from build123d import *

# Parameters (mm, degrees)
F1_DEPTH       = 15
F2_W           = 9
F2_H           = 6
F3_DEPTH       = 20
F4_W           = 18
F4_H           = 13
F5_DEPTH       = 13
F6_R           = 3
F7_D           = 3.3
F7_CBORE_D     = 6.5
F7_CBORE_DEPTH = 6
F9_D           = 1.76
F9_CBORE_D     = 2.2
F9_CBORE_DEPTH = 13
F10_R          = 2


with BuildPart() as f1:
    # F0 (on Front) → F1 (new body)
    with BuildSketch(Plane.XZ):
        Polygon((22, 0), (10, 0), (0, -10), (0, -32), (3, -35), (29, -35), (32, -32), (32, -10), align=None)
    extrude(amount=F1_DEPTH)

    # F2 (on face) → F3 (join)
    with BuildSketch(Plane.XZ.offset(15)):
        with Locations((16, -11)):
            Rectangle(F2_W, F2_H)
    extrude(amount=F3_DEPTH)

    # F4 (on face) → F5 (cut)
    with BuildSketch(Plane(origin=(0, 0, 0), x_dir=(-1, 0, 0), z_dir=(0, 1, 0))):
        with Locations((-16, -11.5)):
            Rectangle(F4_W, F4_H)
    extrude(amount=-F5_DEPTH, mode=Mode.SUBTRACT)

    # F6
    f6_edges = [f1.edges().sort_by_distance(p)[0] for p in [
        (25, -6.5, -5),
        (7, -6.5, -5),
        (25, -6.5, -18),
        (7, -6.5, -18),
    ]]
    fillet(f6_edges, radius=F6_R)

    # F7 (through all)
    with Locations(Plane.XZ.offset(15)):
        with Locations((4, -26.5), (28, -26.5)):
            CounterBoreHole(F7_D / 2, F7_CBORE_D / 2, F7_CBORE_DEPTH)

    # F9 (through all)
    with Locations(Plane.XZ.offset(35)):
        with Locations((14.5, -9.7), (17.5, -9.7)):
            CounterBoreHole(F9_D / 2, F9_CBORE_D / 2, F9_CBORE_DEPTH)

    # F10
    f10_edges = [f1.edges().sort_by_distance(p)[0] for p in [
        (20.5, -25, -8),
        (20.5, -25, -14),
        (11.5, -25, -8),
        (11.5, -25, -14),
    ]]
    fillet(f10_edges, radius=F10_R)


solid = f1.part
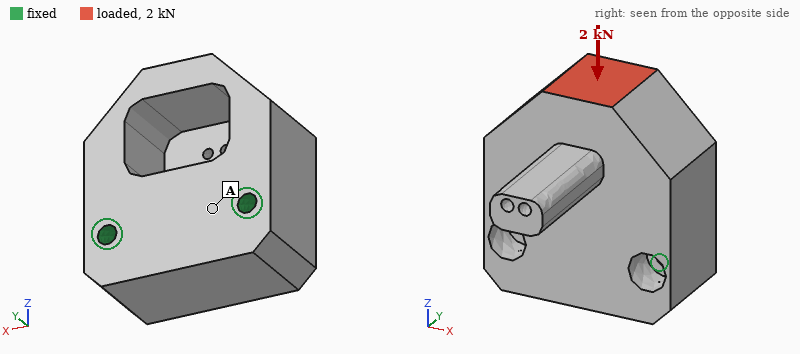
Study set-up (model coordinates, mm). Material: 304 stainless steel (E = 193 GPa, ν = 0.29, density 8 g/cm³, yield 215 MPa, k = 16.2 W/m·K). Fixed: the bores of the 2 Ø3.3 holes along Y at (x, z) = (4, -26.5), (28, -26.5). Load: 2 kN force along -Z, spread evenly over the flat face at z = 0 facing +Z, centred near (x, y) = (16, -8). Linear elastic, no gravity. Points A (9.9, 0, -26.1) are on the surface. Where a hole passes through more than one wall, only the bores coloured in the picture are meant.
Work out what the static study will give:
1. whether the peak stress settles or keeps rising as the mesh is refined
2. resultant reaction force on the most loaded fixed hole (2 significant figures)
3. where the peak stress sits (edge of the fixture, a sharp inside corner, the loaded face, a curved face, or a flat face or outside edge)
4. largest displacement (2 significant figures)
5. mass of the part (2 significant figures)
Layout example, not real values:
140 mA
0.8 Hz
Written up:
keeps rising
1.0 kN
a sharp inside corner
8.0 µm
100 g
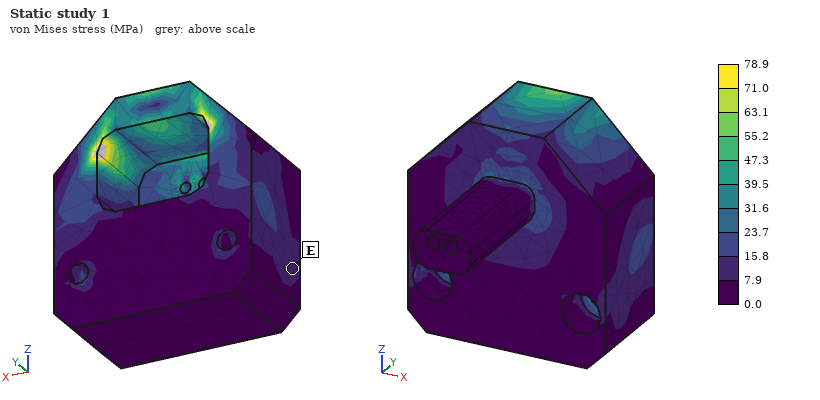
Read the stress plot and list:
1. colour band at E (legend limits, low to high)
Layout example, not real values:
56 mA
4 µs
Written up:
7.9 to 15.8 MPa
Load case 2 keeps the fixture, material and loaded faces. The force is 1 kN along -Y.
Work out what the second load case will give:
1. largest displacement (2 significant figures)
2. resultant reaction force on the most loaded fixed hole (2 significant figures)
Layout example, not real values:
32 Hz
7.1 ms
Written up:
23 µm
510 N
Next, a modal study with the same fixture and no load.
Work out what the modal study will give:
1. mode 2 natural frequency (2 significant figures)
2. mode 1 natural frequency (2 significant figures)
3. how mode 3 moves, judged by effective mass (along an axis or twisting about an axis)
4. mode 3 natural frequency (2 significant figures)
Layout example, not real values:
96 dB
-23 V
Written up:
8800 Hz
6500 Hz
along Y
11 kHz
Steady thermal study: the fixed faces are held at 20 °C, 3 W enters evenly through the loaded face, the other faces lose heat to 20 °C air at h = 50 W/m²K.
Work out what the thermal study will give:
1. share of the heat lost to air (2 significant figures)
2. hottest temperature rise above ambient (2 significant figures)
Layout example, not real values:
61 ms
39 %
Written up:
46 %
23 K
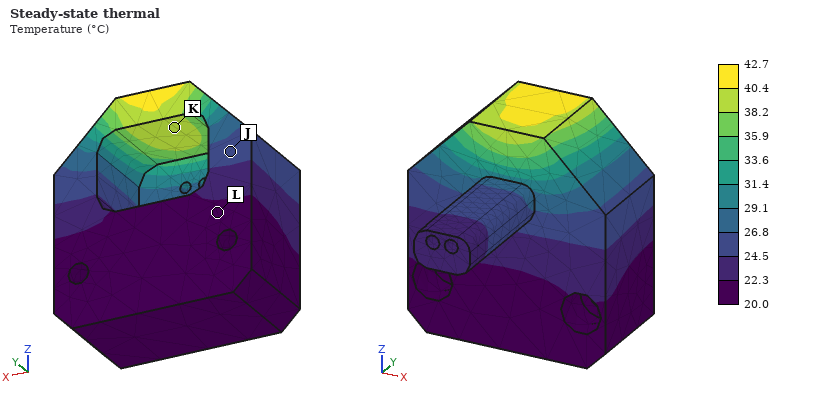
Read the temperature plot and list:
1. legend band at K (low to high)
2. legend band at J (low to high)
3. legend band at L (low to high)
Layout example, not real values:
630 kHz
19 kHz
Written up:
38.2 to 40.4 °C
24.5 to 26.8 °C
20.0 to 22.3 °C
